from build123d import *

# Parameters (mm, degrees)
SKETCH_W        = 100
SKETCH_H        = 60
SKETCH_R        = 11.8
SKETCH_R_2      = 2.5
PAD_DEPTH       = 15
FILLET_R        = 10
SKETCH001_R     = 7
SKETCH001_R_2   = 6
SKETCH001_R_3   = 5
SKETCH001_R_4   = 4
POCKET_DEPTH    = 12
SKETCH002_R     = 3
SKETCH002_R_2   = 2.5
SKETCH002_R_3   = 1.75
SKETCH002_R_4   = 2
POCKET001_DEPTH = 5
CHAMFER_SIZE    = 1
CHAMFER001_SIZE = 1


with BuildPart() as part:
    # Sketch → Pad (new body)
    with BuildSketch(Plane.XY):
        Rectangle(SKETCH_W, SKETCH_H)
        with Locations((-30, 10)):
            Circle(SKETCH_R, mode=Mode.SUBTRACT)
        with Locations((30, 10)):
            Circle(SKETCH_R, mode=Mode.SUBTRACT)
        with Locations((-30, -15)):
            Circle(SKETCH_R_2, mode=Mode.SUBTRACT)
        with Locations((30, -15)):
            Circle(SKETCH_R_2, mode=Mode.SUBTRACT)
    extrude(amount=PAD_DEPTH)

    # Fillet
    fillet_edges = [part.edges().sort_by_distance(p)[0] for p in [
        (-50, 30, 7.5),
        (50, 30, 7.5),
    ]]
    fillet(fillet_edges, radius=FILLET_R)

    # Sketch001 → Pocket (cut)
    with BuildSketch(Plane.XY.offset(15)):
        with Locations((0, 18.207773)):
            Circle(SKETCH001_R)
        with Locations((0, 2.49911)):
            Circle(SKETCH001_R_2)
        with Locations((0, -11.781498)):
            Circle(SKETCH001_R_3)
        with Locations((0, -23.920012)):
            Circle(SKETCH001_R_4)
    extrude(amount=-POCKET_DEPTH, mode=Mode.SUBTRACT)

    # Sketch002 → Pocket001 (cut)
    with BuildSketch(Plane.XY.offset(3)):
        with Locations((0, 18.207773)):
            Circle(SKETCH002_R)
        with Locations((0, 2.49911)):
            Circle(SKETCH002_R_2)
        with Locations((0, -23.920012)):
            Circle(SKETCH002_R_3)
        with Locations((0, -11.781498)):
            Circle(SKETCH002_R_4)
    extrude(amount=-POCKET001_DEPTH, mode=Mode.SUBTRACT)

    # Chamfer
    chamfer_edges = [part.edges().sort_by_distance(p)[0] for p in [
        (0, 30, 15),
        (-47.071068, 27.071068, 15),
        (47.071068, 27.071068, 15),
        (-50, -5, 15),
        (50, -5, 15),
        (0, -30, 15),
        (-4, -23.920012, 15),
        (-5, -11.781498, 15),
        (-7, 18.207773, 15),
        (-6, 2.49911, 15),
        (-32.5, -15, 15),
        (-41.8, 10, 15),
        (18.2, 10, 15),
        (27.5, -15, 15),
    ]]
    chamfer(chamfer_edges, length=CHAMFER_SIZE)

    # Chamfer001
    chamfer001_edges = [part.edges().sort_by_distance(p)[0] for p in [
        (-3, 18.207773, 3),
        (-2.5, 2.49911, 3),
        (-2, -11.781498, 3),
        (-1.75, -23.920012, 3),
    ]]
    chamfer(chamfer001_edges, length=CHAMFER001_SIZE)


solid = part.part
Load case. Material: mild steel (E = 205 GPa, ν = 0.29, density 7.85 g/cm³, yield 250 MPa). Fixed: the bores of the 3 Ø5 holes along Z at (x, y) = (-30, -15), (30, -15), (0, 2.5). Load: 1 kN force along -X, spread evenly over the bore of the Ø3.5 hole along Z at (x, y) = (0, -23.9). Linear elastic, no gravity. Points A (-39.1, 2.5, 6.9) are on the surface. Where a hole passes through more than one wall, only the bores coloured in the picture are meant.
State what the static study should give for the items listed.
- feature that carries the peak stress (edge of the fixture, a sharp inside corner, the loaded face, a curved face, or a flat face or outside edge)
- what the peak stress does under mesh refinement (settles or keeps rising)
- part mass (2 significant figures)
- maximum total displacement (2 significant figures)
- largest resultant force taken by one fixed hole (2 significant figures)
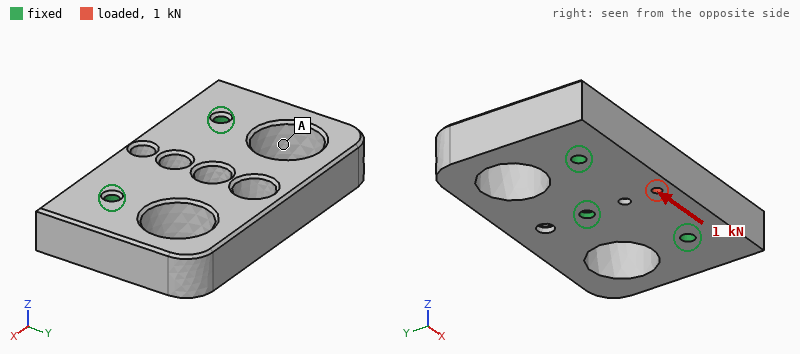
a sharp inside corner
keeps rising
550 g
1.3 µm
510 N
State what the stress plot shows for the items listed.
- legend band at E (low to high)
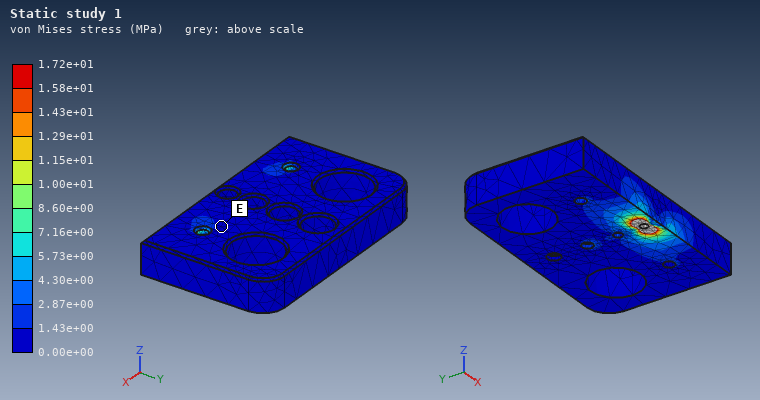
0.00e+00 to 1.43e+00 MPa
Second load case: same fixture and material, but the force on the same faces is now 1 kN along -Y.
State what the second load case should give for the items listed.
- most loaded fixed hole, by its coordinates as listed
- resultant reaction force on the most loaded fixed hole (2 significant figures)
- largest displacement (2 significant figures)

(0, 2.5)
410 N
2.2 µm
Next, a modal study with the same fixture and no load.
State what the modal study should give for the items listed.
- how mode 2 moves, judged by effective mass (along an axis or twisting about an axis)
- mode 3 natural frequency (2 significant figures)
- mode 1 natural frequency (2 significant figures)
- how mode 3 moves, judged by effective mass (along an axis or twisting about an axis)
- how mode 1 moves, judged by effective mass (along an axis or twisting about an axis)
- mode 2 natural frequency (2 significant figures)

twisting about Y
10 kHz
5300 Hz
along X
along Z
6200 Hz
